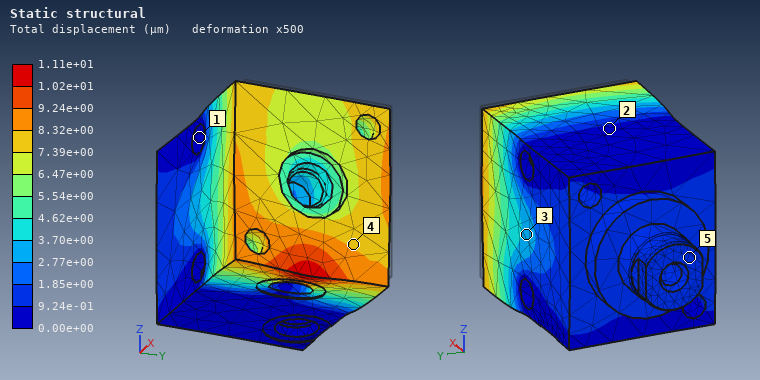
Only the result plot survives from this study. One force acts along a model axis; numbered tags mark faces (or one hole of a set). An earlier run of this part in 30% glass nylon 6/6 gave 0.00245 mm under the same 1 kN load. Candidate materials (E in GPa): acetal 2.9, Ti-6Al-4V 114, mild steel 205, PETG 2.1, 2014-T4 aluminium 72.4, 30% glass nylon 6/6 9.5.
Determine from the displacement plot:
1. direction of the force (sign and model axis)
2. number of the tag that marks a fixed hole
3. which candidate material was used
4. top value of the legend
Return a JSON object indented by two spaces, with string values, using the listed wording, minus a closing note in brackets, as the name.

{
  "direction of the force": "-X",
  "number of the tag that marks a fixed hole": "1",
  "which candidate material was used": "PETG",
  "top value of the legend": "1.11e+01 µm"
}
